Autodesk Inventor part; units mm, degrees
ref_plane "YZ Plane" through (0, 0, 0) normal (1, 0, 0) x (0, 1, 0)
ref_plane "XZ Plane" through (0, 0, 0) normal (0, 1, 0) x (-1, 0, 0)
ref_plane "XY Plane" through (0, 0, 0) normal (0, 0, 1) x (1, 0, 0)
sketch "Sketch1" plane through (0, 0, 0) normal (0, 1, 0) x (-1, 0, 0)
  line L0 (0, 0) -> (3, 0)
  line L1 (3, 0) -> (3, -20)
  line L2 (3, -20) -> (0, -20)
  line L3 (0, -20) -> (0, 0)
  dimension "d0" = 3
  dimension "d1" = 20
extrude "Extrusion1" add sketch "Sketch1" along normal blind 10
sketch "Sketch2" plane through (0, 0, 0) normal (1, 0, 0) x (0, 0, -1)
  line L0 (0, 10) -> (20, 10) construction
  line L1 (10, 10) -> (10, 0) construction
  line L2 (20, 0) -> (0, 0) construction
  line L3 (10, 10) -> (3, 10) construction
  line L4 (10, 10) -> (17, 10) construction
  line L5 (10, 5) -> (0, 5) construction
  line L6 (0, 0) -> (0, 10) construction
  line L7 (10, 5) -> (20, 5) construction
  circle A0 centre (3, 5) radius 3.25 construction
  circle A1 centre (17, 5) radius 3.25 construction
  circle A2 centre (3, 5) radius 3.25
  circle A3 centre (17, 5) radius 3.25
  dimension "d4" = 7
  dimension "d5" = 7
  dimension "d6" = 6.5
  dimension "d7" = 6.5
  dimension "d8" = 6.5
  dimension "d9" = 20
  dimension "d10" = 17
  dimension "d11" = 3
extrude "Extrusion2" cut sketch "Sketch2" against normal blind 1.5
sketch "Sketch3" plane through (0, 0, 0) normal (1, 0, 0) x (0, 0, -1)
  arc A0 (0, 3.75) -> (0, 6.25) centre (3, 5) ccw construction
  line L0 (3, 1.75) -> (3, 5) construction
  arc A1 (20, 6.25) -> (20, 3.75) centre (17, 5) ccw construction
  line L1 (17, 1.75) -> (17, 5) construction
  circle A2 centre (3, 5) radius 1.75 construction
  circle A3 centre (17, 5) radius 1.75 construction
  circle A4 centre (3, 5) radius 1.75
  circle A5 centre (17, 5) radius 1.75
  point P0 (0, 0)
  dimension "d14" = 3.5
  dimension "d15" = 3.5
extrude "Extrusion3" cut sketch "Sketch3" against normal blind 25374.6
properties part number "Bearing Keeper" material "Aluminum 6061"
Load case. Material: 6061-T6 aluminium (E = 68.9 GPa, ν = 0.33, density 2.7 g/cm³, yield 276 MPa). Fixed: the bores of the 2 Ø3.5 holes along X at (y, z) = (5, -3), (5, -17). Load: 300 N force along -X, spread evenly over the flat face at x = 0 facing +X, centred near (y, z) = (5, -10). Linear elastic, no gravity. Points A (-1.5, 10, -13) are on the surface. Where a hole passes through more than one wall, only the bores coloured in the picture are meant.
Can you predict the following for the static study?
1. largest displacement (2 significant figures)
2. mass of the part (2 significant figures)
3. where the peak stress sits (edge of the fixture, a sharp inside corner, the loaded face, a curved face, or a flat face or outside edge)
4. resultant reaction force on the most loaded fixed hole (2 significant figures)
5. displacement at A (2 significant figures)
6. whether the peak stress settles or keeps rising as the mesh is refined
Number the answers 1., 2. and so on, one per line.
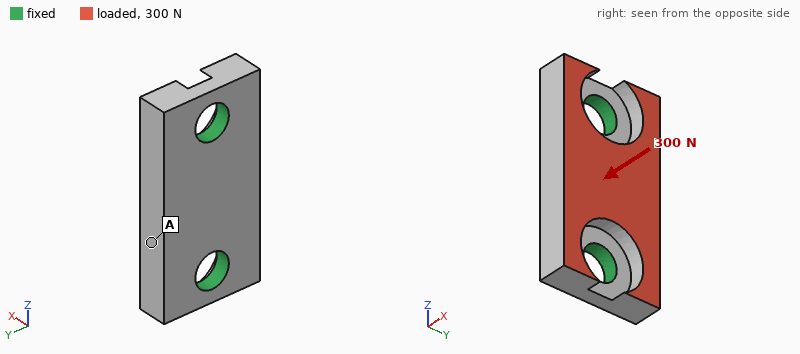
1. 3.7 µm
2. 1.3 g
3. edge of the fixture
4. 160 N
5. 3.2 µm
6. keeps rising
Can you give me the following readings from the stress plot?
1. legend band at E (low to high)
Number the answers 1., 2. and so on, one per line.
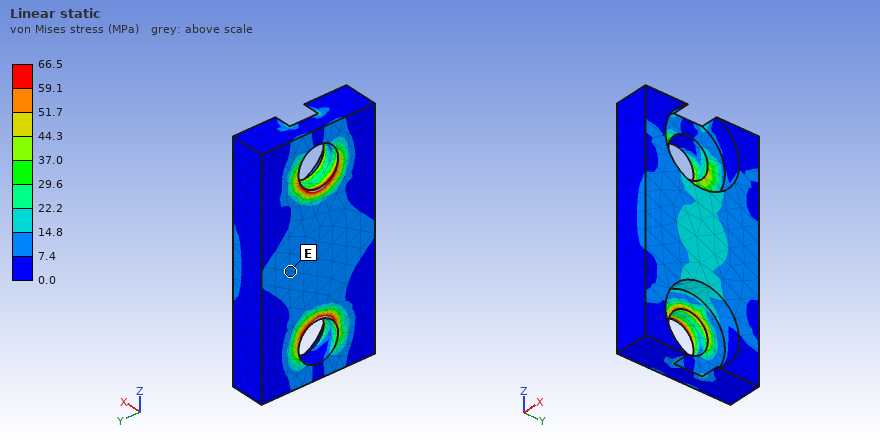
1. 7.4 to 14.8 MPa
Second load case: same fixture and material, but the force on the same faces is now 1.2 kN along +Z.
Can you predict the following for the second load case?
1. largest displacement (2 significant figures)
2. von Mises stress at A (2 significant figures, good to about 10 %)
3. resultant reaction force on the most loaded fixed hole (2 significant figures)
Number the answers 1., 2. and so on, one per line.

1. 7.4 µm
2. 10 MPa
3. 630 N
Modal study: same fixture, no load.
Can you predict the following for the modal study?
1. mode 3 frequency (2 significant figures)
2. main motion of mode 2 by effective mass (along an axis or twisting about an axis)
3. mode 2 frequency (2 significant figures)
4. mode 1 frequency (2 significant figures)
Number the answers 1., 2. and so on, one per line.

1. 70 kHz
2. along X
3. 51 kHz
4. 39 kHz
